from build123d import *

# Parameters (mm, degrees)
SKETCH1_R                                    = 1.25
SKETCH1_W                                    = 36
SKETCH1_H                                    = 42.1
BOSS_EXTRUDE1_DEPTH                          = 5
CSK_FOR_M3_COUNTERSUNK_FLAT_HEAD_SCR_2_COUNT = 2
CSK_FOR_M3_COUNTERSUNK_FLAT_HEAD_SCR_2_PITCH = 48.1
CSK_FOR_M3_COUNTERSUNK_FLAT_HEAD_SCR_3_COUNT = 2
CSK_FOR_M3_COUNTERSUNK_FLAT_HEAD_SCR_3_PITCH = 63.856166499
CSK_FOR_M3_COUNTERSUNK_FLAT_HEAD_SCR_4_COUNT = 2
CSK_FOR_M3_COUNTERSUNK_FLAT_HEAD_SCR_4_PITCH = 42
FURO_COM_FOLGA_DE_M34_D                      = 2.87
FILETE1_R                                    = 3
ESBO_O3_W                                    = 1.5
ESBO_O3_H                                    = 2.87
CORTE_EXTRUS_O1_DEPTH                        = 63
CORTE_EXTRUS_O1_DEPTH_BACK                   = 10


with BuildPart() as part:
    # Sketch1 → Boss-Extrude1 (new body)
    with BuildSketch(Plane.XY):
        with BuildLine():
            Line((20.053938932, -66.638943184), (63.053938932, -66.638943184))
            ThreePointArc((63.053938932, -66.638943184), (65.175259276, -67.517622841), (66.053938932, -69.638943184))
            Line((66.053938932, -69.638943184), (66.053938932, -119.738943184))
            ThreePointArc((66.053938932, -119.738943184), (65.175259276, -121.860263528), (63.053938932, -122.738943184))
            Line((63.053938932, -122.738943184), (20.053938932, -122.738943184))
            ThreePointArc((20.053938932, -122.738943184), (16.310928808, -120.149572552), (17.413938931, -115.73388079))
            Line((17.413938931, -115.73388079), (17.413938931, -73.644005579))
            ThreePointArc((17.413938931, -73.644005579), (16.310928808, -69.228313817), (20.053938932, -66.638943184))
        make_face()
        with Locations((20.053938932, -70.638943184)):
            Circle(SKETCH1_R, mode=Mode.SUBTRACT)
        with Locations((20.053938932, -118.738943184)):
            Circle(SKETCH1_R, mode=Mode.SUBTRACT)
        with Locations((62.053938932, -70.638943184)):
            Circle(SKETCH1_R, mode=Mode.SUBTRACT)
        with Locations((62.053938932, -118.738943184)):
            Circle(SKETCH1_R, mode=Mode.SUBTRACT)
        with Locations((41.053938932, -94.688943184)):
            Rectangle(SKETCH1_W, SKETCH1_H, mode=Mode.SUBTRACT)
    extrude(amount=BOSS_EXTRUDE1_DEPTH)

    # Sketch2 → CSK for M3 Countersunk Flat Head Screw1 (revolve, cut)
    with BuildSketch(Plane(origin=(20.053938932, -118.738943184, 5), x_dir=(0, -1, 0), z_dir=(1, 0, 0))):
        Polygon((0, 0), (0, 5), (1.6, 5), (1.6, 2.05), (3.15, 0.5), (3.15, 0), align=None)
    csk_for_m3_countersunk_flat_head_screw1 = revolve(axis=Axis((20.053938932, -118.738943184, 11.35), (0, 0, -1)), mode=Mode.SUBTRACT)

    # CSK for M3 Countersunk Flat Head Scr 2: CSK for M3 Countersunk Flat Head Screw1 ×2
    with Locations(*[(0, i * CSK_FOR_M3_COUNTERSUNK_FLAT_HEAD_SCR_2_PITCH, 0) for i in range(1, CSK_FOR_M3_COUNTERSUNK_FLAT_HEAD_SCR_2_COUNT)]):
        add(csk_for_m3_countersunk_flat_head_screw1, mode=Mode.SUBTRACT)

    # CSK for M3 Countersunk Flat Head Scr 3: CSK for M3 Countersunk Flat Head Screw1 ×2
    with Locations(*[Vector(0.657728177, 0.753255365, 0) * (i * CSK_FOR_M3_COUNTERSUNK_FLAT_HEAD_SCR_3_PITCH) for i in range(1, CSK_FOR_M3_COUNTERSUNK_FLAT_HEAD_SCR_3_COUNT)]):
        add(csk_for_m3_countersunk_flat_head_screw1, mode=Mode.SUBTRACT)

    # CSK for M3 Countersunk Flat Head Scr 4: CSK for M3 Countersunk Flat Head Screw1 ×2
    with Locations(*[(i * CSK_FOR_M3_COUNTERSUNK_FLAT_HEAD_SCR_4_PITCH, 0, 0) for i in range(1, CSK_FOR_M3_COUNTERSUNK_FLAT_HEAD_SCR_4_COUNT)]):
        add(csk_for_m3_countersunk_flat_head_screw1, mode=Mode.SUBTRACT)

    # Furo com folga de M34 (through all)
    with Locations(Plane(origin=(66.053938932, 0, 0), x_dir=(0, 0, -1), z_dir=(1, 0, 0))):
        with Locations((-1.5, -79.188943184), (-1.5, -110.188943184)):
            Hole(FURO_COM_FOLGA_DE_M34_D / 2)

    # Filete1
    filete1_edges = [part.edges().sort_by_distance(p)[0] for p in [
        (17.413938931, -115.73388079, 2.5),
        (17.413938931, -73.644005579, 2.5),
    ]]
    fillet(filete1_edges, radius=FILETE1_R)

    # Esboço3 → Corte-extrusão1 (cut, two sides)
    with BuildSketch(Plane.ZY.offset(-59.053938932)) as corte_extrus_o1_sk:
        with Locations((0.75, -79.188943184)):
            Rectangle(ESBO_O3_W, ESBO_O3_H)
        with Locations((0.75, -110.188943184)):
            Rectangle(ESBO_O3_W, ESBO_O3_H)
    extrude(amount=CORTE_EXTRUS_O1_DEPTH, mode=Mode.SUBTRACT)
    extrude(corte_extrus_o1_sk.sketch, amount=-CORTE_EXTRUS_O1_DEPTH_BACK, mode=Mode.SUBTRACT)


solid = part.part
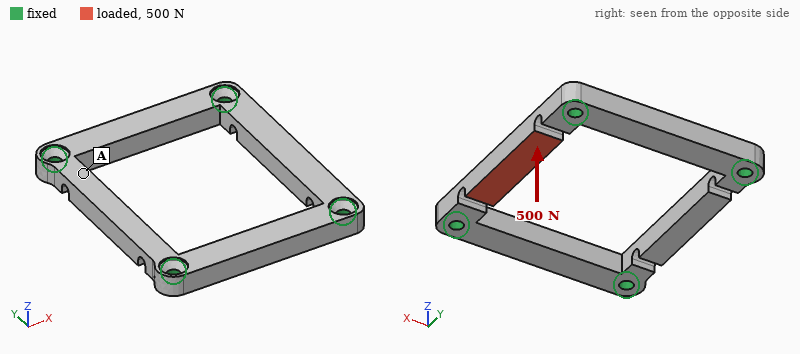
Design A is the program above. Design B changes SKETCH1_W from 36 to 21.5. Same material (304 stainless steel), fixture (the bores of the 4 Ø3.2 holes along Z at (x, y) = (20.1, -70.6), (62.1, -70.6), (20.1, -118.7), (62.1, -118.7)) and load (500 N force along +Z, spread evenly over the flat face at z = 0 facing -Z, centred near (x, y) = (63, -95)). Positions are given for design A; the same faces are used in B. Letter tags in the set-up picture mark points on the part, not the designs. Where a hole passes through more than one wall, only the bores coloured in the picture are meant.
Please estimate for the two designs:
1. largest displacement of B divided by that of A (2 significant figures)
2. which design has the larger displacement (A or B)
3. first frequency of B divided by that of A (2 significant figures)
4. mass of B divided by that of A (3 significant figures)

0.66
A
0.85
1.50
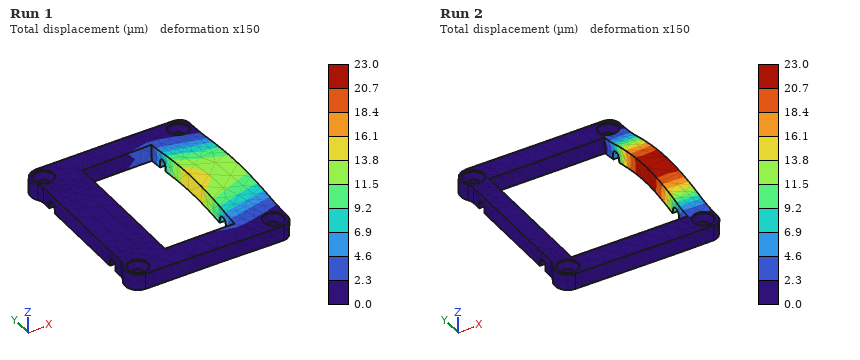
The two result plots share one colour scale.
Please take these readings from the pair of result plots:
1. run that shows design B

Run 1
